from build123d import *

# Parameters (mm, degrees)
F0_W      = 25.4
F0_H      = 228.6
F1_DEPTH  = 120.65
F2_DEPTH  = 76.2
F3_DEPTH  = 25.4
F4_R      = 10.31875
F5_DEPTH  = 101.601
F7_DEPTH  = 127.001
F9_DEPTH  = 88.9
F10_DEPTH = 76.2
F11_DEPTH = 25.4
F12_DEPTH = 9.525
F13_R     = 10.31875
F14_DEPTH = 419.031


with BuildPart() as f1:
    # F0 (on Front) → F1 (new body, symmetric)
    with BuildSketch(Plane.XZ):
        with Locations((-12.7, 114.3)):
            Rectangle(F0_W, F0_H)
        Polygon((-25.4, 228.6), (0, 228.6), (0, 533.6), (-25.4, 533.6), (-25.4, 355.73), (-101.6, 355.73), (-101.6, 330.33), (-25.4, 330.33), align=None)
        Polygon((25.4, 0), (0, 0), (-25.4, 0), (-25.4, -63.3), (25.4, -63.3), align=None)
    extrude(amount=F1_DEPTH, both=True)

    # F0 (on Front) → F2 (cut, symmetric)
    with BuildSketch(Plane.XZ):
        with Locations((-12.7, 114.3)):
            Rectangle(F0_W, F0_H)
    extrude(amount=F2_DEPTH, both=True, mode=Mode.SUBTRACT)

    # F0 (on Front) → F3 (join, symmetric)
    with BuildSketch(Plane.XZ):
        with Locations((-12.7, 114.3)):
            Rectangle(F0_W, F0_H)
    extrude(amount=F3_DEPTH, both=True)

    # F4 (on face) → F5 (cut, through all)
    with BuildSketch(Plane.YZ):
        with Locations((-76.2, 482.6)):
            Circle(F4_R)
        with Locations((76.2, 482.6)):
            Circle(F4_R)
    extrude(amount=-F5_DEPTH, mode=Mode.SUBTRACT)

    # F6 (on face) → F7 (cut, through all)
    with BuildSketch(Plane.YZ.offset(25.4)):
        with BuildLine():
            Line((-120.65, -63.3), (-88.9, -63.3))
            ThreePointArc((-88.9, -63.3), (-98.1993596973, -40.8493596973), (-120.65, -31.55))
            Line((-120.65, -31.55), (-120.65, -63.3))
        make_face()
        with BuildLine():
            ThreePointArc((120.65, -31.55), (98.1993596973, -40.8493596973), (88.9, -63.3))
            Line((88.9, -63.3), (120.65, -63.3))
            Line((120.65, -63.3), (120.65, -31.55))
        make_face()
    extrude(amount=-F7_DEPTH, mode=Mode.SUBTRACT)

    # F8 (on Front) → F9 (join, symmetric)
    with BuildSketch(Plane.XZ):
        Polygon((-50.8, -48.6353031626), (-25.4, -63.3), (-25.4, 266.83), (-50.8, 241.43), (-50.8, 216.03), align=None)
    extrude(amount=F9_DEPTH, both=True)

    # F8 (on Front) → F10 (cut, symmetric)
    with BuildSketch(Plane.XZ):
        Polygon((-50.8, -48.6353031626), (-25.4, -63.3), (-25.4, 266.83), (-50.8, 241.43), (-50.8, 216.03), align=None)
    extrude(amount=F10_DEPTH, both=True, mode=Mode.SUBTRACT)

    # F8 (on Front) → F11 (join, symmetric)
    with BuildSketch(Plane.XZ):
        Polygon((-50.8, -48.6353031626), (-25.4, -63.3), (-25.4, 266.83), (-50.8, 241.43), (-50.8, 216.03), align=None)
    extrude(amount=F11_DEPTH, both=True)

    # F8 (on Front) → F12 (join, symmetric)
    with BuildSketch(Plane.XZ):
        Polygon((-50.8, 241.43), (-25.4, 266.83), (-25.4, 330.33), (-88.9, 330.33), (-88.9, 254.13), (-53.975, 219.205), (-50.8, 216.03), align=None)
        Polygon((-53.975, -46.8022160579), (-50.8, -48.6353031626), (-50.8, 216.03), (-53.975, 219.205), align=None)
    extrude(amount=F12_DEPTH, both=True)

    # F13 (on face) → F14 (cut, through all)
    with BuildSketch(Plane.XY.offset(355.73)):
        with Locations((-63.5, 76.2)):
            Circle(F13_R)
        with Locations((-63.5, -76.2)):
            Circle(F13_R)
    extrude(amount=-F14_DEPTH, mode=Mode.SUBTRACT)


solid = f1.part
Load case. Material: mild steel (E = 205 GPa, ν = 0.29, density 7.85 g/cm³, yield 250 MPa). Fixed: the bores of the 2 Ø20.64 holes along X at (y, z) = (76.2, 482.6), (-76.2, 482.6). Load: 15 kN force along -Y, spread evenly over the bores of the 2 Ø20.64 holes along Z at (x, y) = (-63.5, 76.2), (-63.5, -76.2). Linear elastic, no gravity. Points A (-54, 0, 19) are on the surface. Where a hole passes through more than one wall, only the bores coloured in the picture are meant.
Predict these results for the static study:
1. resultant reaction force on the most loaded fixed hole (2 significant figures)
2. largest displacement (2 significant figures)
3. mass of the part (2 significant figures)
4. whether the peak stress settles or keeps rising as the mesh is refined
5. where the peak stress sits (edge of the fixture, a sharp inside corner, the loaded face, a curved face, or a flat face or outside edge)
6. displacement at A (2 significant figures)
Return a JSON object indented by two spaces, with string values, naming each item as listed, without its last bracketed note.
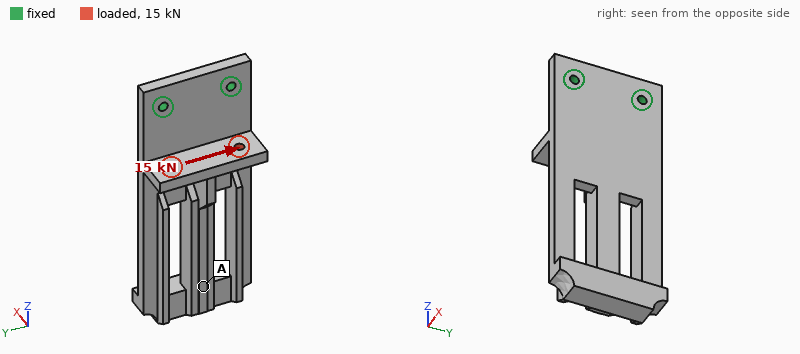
{
  "resultant reaction force on the most loaded fixed hole": "15 kN",
  "largest displacement": "73 µm",
  "mass of the part": "36 kg",
  "whether the peak stress settles or keeps rising as the mesh is refined": "keeps rising",
  "where the peak stress sits": "edge of the fixture",
  "displacement at A": "39 µm"
}
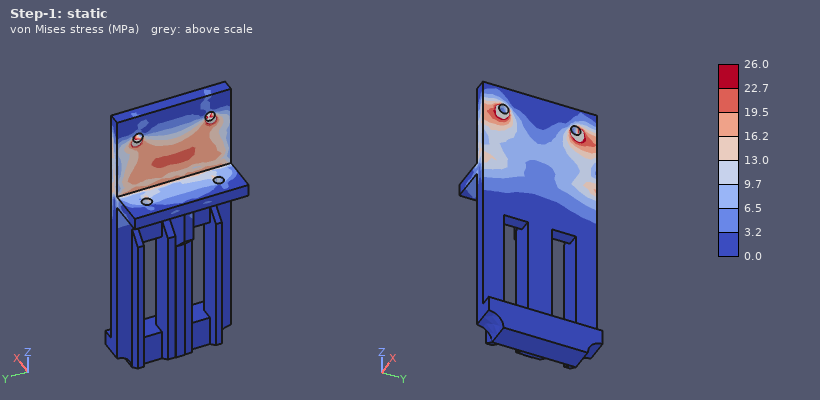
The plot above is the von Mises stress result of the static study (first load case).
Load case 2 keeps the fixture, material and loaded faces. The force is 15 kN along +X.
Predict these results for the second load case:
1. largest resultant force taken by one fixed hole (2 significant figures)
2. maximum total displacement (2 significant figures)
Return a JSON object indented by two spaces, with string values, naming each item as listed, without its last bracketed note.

{
  "largest resultant force taken by one fixed hole": "7.5 kN",
  "maximum total displacement": "1.1 mm"
}
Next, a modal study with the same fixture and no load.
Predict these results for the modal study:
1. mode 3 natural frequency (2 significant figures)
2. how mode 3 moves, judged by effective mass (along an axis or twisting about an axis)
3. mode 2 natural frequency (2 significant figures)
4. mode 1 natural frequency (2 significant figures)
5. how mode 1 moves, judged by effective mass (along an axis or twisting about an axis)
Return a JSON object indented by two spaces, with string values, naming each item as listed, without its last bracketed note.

{
  "mode 3 natural frequency": "370 Hz",
  "how mode 3 moves, judged by effective mass": "along Y",
  "mode 2 natural frequency": "340 Hz",
  "mode 1 natural frequency": "67 Hz",
  "how mode 1 moves, judged by effective mass": "along X"
}
